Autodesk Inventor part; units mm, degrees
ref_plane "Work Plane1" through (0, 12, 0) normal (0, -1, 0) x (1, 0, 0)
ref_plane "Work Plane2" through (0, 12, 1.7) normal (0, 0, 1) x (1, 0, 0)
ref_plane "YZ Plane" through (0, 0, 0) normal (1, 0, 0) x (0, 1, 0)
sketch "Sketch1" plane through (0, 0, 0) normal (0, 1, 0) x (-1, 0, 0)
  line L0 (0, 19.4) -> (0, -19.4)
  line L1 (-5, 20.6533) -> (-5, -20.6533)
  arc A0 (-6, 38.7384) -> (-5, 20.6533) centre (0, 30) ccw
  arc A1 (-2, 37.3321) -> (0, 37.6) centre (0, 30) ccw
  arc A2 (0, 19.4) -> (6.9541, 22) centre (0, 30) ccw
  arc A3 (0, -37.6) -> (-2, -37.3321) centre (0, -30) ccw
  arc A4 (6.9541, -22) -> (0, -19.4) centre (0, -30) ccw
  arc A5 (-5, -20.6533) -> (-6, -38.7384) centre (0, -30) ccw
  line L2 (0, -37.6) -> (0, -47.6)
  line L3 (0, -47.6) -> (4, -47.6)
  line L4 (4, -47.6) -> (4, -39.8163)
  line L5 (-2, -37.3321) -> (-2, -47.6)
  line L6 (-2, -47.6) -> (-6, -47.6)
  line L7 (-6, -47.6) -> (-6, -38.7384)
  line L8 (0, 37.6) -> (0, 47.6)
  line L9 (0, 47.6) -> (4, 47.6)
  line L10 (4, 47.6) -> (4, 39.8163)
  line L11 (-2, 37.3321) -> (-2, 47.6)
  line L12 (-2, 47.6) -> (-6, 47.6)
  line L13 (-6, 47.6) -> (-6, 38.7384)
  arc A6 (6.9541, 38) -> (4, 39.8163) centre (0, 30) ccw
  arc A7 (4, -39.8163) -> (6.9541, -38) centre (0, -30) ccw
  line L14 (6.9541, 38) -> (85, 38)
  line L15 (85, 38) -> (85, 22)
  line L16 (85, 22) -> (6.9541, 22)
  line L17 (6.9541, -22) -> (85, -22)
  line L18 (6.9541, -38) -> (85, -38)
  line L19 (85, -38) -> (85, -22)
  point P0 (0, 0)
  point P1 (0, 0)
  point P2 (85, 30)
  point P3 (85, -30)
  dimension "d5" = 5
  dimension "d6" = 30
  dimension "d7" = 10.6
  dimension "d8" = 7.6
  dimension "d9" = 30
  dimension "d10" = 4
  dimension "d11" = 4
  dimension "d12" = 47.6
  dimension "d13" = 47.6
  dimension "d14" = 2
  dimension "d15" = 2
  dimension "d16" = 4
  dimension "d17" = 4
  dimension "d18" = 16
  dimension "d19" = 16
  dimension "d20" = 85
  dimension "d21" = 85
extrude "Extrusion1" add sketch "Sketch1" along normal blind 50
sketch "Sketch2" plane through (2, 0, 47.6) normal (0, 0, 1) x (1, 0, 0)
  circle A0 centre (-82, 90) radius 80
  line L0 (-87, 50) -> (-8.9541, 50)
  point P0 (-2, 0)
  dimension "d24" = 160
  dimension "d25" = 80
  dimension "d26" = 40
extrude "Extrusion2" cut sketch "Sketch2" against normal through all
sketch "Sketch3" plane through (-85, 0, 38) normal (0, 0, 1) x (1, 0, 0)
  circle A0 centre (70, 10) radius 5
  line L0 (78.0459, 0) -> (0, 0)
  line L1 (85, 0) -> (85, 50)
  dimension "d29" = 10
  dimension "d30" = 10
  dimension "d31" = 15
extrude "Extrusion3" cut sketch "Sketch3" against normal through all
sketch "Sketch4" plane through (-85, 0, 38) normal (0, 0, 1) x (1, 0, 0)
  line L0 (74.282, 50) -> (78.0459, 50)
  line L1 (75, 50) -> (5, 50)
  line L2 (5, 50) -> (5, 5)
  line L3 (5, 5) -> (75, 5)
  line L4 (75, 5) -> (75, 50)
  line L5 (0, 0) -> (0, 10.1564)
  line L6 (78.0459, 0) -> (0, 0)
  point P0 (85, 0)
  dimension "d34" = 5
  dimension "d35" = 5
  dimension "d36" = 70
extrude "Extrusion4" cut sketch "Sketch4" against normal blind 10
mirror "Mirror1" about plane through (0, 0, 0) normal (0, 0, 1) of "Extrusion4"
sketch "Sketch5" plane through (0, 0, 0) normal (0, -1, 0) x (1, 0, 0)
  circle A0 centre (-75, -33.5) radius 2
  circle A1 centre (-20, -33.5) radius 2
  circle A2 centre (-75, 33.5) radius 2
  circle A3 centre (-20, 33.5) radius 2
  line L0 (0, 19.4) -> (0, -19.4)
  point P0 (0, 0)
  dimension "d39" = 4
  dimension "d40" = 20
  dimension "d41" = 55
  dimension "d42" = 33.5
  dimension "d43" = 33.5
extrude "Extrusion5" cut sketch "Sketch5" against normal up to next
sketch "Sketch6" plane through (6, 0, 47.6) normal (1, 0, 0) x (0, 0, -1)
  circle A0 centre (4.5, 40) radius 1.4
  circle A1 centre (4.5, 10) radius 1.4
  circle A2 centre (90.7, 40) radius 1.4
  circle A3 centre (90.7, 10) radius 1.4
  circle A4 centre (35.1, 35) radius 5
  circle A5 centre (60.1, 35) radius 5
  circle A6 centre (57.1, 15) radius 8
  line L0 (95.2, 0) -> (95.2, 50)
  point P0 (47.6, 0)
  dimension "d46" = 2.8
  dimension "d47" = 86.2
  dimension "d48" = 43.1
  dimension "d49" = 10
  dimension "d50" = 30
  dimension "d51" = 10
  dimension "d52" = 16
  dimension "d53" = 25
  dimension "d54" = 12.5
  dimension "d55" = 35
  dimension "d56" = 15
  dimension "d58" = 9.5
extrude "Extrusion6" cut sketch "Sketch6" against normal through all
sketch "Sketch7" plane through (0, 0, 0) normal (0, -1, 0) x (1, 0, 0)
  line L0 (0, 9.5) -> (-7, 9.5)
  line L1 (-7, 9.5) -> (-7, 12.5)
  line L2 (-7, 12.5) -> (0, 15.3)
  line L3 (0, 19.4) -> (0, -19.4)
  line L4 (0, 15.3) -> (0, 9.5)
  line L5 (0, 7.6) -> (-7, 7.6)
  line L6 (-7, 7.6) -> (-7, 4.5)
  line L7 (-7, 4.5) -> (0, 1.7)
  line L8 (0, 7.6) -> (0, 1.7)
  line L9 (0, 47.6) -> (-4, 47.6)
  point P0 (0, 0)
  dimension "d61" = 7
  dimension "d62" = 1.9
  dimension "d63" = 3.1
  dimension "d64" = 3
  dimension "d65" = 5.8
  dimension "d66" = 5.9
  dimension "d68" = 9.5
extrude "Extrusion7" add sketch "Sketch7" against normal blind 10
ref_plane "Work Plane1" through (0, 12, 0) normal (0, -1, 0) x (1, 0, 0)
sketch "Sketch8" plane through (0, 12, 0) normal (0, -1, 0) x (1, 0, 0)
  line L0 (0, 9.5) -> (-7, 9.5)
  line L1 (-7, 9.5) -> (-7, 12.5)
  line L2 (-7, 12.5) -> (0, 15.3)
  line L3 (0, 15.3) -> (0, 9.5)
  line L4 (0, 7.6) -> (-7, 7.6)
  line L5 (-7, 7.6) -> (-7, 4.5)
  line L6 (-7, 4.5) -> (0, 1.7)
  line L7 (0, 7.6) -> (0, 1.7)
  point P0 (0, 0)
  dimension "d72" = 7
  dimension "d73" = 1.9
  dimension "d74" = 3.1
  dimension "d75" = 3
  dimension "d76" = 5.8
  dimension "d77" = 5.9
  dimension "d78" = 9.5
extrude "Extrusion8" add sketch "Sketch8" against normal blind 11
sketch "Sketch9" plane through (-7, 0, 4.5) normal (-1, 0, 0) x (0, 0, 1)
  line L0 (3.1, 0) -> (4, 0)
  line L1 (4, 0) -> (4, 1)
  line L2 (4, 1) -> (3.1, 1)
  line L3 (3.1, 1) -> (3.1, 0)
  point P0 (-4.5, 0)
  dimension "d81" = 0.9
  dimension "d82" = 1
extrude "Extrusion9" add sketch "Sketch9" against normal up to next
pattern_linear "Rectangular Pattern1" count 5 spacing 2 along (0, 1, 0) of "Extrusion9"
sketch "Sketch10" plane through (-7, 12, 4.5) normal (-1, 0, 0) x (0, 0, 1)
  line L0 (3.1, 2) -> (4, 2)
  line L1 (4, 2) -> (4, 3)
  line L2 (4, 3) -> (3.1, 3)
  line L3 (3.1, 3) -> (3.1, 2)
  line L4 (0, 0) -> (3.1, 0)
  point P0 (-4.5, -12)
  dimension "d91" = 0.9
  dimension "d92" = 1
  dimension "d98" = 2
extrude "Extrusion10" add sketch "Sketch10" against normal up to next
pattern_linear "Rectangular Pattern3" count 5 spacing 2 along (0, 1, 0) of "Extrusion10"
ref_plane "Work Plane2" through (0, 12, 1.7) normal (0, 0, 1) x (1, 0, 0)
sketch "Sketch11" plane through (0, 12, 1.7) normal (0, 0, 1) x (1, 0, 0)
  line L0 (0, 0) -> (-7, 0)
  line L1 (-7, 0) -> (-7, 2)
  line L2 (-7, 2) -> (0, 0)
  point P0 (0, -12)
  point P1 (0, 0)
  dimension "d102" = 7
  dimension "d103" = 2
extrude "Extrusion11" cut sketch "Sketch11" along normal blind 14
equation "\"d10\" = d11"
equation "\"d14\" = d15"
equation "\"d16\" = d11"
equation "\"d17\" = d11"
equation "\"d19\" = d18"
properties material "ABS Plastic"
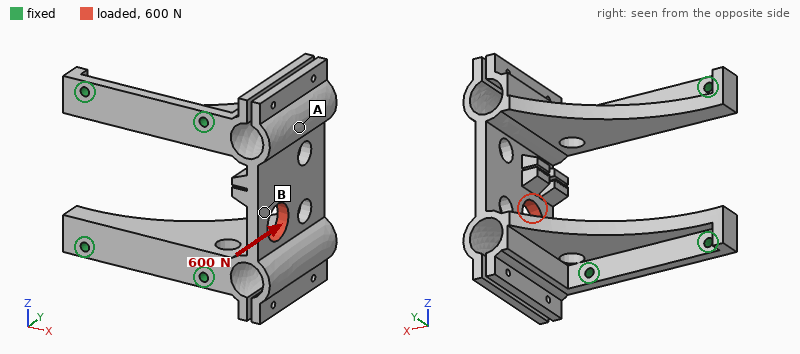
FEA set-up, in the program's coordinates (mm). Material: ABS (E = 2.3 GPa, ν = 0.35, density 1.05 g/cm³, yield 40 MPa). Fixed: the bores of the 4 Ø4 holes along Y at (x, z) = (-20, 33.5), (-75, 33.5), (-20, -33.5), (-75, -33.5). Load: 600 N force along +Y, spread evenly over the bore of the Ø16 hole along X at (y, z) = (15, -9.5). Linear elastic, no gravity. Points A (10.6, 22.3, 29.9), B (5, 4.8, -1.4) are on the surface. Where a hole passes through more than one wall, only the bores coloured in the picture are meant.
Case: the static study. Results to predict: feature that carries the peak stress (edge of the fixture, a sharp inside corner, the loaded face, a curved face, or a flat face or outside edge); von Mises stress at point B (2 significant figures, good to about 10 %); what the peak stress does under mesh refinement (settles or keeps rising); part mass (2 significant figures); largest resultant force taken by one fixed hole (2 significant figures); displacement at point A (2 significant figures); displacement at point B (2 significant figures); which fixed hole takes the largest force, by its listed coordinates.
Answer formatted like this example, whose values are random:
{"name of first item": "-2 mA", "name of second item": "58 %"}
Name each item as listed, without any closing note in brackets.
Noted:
{"feature that carries the peak stress": "edge of the fixture", "von Mises stress at point B": "5.7 MPa", "what the peak stress does under mesh refinement": "keeps rising", "part mass": "61 g", "largest resultant force taken by one fixed hole": "540 N", "displacement at point A": "0.41 mm", "displacement at point B": "0.55 mm", "which fixed hole takes the largest force, by its listed coordinates": "(-20, -33.5)"}
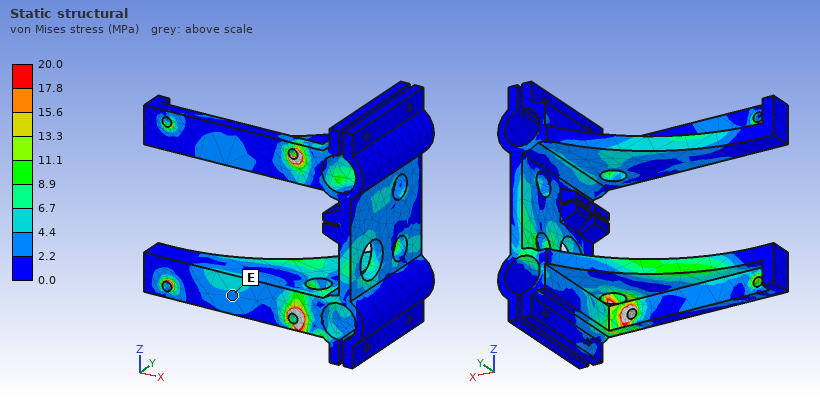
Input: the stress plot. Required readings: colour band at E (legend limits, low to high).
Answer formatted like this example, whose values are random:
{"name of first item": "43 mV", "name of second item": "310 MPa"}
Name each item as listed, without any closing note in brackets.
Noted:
{"colour band at E": "2.2 to 4.4 MPa"}
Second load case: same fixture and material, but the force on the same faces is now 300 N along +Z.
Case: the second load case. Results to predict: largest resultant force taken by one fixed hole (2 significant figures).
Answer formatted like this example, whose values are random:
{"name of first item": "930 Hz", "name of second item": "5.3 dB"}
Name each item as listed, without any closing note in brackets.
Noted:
{"largest resultant force taken by one fixed hole": "220 N"}
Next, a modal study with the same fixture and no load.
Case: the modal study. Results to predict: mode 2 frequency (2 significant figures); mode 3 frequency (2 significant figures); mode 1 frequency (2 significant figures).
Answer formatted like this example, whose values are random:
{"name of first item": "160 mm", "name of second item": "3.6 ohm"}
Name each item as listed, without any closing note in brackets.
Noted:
{"mode 2 frequency": "690 Hz", "mode 3 frequency": "810 Hz", "mode 1 frequency": "670 Hz"}
